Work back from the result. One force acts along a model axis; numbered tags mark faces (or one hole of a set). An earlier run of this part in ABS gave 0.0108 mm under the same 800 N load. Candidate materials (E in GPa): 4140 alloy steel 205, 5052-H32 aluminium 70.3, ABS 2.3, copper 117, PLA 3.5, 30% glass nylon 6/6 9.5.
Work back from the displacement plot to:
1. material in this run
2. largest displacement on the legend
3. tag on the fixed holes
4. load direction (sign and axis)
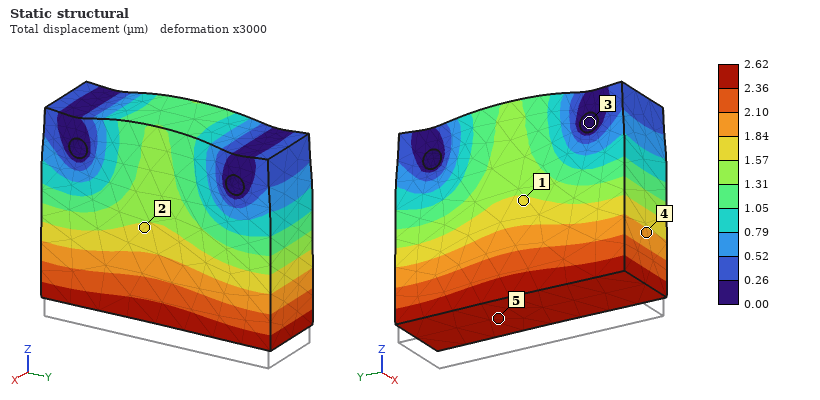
30% glass nylon 6/6
2.62 µm
3
+Z
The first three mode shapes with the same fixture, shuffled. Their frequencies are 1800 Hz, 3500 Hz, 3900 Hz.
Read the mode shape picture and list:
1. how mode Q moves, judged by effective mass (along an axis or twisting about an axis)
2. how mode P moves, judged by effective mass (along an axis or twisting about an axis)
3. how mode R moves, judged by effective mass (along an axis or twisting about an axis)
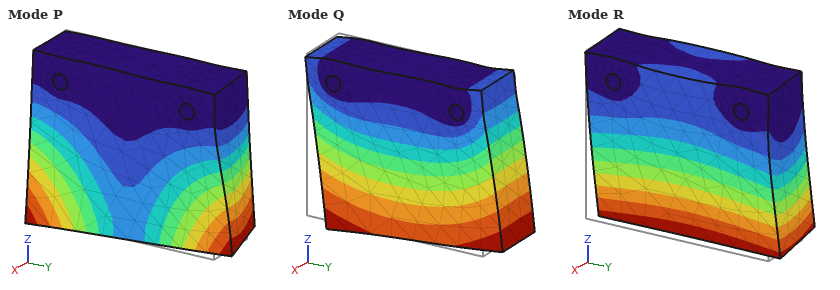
along Y
twisting about Z
along X
